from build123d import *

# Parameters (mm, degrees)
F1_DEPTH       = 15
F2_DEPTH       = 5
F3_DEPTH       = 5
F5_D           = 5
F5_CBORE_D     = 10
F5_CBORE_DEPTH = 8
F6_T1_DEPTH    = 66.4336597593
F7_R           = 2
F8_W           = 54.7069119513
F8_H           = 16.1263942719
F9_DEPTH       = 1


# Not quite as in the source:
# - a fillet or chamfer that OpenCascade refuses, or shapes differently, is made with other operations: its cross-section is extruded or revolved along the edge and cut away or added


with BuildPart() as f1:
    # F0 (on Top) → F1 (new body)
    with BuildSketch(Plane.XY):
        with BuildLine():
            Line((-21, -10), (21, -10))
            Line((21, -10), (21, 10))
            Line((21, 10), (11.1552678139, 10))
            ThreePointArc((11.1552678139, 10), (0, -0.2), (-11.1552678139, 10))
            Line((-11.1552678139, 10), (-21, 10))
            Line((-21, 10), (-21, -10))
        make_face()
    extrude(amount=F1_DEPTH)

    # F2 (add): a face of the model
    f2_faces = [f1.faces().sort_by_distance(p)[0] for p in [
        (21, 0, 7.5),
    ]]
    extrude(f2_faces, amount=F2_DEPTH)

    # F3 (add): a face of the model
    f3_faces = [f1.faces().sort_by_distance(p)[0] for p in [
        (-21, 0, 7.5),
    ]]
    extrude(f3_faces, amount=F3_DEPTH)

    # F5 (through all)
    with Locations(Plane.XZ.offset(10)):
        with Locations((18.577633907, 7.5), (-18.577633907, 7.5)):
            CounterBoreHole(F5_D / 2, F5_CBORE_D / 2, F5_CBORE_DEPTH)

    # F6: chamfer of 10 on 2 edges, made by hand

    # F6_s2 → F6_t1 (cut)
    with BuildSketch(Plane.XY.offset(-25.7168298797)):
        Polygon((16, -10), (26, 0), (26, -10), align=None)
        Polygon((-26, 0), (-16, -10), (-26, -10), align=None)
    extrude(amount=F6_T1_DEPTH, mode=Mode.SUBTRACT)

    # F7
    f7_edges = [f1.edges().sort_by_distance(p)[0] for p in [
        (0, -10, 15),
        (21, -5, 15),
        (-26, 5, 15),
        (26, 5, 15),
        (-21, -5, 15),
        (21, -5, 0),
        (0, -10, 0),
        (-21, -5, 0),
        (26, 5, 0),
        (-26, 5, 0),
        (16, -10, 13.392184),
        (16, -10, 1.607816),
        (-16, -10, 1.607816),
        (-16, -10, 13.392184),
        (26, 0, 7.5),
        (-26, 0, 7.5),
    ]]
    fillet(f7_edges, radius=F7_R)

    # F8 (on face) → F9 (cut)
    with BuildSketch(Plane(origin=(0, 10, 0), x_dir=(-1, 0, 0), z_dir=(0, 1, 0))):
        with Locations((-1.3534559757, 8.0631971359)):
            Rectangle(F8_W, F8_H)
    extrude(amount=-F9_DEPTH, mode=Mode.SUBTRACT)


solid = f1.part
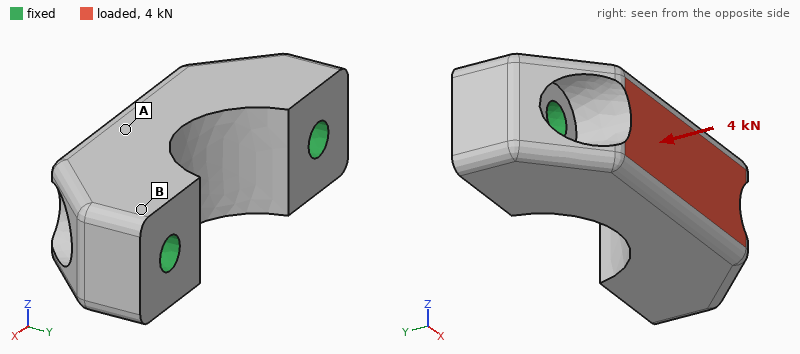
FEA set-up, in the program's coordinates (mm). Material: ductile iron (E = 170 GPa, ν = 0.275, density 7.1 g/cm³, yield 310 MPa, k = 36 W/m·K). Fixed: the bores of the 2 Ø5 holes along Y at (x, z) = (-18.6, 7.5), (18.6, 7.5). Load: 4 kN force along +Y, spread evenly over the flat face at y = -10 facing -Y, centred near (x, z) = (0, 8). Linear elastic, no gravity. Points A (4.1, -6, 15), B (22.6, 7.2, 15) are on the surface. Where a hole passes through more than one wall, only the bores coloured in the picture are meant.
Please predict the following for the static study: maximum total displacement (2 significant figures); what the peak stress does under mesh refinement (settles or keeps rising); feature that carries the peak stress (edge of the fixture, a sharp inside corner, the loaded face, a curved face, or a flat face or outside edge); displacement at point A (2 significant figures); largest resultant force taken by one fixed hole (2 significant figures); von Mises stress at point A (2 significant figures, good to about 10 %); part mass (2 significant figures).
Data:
3.4 µm
keeps rising
edge of the fixture
2.9 µm
2.4 kN
11 MPa
68 g
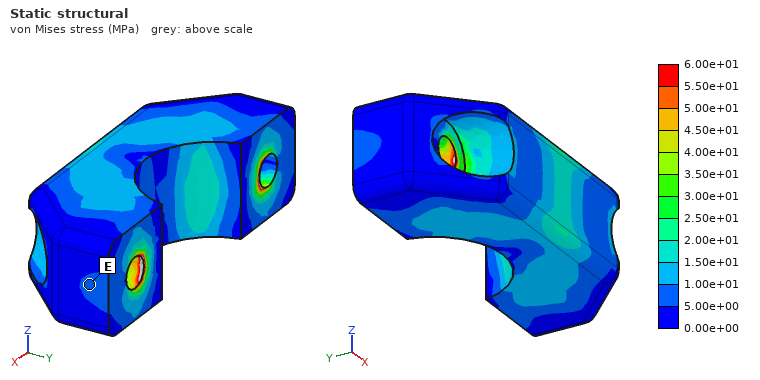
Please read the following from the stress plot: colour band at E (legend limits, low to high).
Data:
5.00e+00 to 1.00e+01 MPa
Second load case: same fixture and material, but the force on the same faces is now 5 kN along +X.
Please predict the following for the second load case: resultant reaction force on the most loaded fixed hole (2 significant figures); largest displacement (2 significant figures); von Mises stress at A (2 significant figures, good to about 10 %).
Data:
3.0 kN
4.2 µm
20 MPa
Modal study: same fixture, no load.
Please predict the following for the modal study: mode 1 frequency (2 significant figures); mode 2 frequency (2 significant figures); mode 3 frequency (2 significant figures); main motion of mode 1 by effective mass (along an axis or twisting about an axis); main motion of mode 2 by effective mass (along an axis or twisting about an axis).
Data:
20 kHz
33 kHz
40 kHz
along Z
along Y
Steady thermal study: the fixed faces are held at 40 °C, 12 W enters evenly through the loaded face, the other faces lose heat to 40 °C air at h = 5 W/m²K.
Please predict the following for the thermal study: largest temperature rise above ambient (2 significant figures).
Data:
18 K
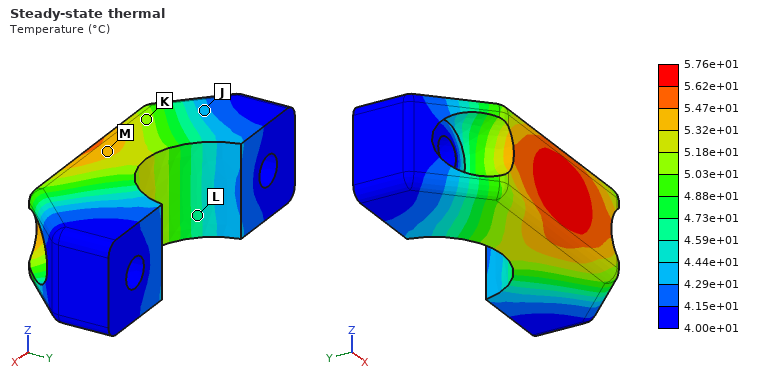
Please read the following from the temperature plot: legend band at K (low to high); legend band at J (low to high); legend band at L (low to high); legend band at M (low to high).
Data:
5.03e+01 to 5.18e+01 °C
4.29e+01 to 4.44e+01 °C
4.59e+01 to 4.73e+01 °C
5.32e+01 to 5.47e+01 °C
